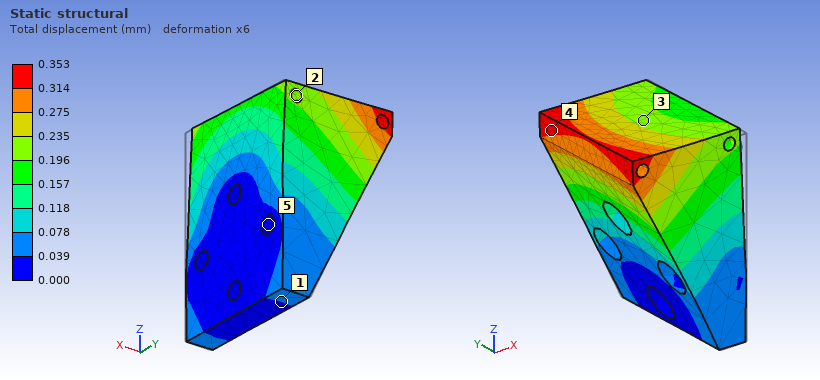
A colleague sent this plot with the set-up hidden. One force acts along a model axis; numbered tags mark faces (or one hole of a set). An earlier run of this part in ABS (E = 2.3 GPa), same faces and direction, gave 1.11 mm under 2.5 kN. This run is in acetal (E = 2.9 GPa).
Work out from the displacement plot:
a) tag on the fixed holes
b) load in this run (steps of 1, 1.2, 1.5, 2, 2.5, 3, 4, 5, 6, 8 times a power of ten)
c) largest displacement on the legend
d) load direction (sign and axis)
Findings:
5
1 kN
0.353 mm
+Y
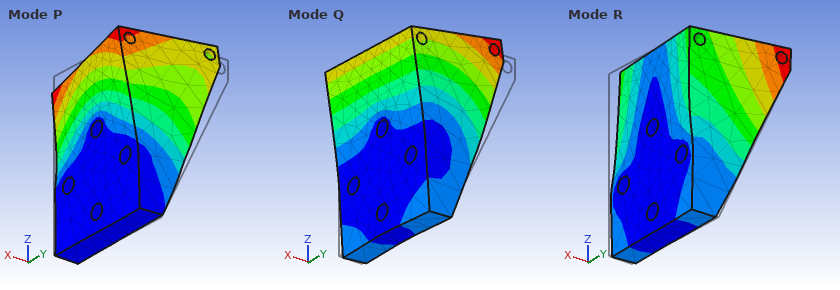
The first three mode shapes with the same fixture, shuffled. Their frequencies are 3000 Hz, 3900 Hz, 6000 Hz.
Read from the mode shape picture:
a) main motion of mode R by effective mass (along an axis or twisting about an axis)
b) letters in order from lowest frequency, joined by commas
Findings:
along Y
Q, R, P
